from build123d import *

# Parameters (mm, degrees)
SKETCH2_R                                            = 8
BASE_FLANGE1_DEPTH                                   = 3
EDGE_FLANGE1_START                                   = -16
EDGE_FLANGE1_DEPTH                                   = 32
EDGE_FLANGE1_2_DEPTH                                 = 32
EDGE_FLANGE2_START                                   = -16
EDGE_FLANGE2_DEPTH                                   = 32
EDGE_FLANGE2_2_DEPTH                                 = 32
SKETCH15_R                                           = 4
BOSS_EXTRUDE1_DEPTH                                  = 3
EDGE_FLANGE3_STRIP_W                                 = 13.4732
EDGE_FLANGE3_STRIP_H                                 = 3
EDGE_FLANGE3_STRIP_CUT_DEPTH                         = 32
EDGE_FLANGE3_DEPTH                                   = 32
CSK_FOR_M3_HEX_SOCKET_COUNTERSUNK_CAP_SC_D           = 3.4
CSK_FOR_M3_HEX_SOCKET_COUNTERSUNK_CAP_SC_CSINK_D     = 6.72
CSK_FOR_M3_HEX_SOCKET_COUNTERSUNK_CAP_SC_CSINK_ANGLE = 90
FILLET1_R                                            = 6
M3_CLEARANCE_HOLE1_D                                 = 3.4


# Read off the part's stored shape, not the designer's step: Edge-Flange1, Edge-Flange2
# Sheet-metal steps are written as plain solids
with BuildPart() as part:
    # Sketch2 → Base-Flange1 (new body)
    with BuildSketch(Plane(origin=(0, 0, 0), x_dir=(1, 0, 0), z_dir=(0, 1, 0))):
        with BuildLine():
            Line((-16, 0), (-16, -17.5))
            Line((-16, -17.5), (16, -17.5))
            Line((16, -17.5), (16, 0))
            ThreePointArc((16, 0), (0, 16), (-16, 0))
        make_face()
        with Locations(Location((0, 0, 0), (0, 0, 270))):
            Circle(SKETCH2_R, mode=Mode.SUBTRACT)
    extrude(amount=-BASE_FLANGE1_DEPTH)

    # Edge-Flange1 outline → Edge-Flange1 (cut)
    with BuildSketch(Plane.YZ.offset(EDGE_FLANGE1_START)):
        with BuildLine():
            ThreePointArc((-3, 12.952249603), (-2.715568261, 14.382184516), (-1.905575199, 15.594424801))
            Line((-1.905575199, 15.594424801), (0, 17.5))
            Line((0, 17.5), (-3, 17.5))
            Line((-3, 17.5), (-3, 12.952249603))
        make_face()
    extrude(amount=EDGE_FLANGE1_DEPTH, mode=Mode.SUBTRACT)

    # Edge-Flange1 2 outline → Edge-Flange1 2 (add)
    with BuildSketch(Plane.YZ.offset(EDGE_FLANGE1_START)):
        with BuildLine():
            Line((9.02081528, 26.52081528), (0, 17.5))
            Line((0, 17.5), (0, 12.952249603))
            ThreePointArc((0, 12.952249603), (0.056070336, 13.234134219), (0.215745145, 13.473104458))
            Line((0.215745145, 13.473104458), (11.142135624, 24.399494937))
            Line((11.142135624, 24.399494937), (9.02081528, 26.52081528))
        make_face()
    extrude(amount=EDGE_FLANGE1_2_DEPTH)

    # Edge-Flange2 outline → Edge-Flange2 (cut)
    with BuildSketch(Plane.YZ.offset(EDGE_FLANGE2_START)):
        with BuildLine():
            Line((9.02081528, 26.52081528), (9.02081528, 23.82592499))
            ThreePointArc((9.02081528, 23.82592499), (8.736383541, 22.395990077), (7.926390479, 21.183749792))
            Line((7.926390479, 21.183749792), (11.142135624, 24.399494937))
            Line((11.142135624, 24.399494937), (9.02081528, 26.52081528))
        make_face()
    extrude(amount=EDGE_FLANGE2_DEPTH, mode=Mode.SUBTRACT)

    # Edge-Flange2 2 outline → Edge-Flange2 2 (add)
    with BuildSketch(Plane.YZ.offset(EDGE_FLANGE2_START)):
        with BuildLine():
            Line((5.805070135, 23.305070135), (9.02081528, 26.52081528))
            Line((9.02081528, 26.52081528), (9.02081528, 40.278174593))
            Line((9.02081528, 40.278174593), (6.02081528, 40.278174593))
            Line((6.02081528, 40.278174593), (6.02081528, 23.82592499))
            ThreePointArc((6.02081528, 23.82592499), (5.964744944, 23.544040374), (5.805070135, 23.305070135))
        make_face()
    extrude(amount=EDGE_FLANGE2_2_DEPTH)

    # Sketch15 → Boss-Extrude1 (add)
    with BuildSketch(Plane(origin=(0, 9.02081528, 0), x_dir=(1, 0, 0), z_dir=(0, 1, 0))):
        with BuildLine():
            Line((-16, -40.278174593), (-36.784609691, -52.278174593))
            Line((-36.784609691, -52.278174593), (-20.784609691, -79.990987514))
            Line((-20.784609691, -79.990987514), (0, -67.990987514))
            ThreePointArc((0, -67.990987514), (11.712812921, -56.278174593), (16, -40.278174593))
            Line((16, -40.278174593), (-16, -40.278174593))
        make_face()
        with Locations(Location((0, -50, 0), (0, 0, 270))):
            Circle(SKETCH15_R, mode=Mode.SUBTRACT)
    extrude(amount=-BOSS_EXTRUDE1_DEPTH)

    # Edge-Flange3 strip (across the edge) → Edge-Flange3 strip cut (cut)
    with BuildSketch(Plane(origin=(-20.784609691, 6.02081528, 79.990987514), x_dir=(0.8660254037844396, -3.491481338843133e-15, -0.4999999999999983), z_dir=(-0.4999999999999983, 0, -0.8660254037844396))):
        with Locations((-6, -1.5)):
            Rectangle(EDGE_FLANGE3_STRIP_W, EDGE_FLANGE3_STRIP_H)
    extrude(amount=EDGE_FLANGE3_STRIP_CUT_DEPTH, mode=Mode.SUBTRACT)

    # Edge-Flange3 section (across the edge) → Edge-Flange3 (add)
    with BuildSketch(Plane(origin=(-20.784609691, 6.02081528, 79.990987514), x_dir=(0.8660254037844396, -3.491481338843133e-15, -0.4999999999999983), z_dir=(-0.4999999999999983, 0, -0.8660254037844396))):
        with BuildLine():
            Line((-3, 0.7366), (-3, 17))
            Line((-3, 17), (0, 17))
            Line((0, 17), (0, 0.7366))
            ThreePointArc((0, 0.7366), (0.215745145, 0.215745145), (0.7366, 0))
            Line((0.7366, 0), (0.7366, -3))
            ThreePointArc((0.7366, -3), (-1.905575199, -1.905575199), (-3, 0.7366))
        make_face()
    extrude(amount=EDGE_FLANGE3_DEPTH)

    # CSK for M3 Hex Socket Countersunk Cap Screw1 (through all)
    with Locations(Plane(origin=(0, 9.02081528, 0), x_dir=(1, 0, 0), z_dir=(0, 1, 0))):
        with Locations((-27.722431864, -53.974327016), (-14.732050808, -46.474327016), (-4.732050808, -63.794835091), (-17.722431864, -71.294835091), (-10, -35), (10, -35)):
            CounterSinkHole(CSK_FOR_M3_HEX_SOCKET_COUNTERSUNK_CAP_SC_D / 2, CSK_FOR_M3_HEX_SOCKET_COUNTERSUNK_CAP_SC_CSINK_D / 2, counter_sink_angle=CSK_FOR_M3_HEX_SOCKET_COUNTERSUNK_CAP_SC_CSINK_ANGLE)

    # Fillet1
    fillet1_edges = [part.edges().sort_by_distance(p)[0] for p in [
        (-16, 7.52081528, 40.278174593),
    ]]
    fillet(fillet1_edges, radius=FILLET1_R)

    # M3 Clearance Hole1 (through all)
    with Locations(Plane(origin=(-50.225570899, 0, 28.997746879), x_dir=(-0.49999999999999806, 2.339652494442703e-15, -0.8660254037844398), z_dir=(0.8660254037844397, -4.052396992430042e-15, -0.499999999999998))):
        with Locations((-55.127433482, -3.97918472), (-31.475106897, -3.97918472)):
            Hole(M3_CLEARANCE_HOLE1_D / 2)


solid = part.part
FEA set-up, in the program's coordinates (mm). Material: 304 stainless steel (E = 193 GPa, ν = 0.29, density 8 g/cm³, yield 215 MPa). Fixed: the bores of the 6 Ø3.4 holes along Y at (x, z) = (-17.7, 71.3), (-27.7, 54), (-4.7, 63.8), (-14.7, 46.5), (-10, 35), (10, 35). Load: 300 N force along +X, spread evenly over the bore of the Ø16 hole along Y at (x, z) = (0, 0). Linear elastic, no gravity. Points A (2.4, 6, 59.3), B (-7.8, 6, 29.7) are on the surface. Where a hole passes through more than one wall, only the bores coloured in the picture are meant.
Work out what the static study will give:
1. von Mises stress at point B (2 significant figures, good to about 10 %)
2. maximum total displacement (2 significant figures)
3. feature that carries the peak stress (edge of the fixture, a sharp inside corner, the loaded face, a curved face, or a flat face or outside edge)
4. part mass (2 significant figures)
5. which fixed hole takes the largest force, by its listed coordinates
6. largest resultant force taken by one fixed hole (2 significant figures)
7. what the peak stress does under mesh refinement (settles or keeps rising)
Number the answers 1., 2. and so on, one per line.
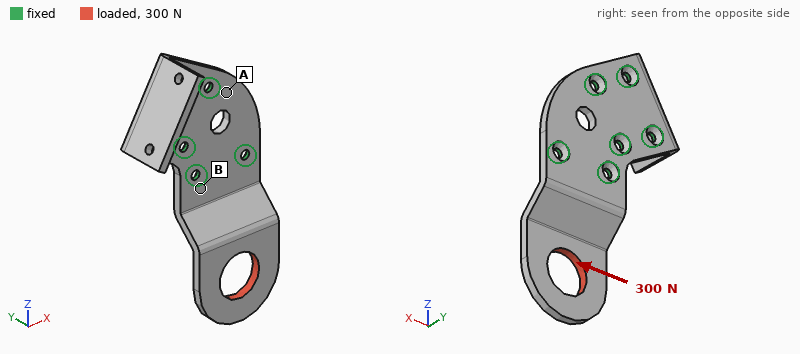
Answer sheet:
1. 30 MPa
2. 28 µm
3. edge of the fixture
4. 81 g
5. (10, 35)
6. 440 N
7. keeps rising
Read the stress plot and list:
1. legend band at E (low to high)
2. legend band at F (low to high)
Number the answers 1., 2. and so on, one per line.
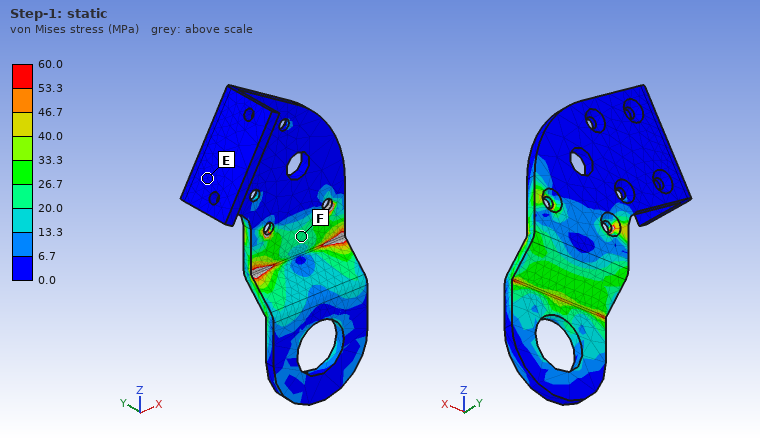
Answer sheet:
1. 0.0 to 6.7 MPa
2. 20.0 to 26.7 MPa
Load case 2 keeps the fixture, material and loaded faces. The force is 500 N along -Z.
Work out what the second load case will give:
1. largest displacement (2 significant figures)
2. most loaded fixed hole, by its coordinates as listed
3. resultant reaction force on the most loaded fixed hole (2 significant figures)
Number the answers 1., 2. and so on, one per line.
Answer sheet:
1. 0.28 mm
2. (-10, 35)
3. 410 N
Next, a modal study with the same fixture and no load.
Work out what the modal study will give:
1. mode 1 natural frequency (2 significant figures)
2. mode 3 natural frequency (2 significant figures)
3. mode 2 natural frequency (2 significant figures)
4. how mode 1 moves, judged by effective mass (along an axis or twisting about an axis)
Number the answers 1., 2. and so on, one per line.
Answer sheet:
1. 990 Hz
2. 3800 Hz
3. 3300 Hz
4. along Y
